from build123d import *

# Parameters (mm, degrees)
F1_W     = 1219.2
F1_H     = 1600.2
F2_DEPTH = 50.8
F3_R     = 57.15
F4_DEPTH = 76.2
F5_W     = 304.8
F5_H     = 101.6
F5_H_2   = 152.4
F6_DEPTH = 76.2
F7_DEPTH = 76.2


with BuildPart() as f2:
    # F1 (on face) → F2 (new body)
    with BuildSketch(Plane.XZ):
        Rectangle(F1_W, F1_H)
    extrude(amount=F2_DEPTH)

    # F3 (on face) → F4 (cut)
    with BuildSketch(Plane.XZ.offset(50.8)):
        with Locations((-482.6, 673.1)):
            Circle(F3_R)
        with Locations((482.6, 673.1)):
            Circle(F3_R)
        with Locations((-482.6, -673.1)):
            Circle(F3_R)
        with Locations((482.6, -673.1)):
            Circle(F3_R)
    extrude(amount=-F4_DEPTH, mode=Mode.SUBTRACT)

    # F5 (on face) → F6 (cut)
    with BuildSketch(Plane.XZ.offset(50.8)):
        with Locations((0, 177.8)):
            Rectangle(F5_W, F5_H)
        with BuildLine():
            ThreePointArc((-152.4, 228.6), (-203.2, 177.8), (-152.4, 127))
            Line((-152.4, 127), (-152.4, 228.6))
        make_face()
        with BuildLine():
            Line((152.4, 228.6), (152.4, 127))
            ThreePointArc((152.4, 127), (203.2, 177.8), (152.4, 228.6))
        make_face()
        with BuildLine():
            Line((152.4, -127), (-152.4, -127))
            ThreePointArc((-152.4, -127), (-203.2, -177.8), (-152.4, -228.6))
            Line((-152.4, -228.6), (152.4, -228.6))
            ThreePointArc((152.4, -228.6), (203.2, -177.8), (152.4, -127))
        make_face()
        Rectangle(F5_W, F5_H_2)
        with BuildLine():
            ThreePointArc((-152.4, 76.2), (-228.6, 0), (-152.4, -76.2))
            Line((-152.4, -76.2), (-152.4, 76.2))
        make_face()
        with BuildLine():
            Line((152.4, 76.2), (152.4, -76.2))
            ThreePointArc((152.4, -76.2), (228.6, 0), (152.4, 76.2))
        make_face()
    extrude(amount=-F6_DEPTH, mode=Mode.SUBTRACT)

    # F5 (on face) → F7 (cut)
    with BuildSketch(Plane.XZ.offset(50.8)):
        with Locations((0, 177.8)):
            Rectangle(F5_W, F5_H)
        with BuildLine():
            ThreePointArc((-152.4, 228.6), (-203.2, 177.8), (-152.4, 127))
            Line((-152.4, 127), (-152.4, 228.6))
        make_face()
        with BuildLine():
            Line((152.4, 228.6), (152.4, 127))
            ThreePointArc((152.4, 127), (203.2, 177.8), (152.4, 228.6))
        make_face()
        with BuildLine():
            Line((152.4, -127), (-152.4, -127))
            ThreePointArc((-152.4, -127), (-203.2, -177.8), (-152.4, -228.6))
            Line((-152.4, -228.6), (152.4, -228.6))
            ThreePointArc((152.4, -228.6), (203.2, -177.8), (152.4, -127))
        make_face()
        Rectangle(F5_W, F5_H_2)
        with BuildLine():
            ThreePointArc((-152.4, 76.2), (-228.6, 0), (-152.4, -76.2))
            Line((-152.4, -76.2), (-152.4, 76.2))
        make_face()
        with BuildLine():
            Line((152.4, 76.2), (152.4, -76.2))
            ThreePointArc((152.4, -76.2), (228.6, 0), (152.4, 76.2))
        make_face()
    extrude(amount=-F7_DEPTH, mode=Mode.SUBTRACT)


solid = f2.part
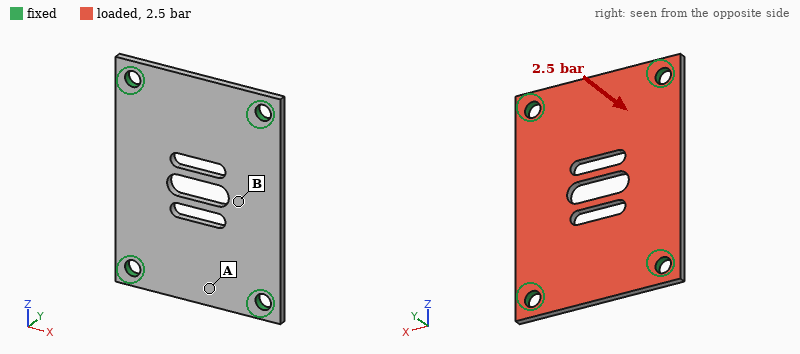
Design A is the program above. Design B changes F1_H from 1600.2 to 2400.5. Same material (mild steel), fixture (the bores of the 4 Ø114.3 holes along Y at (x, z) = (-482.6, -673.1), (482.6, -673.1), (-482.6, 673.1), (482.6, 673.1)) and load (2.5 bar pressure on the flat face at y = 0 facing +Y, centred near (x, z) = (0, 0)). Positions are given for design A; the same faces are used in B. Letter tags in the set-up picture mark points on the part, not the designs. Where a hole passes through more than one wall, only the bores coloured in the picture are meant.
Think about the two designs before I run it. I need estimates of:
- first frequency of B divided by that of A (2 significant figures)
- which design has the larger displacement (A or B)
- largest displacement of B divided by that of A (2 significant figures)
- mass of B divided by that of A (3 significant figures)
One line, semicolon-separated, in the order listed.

0.92; A; 0.85; 1.55
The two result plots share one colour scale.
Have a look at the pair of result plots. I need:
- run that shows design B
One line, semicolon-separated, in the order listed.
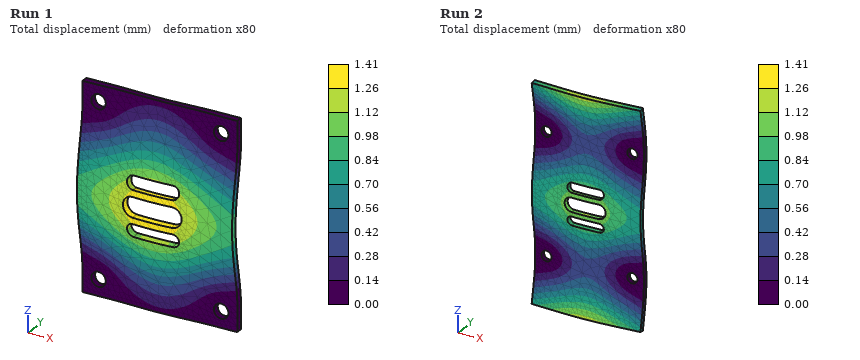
Run 2
